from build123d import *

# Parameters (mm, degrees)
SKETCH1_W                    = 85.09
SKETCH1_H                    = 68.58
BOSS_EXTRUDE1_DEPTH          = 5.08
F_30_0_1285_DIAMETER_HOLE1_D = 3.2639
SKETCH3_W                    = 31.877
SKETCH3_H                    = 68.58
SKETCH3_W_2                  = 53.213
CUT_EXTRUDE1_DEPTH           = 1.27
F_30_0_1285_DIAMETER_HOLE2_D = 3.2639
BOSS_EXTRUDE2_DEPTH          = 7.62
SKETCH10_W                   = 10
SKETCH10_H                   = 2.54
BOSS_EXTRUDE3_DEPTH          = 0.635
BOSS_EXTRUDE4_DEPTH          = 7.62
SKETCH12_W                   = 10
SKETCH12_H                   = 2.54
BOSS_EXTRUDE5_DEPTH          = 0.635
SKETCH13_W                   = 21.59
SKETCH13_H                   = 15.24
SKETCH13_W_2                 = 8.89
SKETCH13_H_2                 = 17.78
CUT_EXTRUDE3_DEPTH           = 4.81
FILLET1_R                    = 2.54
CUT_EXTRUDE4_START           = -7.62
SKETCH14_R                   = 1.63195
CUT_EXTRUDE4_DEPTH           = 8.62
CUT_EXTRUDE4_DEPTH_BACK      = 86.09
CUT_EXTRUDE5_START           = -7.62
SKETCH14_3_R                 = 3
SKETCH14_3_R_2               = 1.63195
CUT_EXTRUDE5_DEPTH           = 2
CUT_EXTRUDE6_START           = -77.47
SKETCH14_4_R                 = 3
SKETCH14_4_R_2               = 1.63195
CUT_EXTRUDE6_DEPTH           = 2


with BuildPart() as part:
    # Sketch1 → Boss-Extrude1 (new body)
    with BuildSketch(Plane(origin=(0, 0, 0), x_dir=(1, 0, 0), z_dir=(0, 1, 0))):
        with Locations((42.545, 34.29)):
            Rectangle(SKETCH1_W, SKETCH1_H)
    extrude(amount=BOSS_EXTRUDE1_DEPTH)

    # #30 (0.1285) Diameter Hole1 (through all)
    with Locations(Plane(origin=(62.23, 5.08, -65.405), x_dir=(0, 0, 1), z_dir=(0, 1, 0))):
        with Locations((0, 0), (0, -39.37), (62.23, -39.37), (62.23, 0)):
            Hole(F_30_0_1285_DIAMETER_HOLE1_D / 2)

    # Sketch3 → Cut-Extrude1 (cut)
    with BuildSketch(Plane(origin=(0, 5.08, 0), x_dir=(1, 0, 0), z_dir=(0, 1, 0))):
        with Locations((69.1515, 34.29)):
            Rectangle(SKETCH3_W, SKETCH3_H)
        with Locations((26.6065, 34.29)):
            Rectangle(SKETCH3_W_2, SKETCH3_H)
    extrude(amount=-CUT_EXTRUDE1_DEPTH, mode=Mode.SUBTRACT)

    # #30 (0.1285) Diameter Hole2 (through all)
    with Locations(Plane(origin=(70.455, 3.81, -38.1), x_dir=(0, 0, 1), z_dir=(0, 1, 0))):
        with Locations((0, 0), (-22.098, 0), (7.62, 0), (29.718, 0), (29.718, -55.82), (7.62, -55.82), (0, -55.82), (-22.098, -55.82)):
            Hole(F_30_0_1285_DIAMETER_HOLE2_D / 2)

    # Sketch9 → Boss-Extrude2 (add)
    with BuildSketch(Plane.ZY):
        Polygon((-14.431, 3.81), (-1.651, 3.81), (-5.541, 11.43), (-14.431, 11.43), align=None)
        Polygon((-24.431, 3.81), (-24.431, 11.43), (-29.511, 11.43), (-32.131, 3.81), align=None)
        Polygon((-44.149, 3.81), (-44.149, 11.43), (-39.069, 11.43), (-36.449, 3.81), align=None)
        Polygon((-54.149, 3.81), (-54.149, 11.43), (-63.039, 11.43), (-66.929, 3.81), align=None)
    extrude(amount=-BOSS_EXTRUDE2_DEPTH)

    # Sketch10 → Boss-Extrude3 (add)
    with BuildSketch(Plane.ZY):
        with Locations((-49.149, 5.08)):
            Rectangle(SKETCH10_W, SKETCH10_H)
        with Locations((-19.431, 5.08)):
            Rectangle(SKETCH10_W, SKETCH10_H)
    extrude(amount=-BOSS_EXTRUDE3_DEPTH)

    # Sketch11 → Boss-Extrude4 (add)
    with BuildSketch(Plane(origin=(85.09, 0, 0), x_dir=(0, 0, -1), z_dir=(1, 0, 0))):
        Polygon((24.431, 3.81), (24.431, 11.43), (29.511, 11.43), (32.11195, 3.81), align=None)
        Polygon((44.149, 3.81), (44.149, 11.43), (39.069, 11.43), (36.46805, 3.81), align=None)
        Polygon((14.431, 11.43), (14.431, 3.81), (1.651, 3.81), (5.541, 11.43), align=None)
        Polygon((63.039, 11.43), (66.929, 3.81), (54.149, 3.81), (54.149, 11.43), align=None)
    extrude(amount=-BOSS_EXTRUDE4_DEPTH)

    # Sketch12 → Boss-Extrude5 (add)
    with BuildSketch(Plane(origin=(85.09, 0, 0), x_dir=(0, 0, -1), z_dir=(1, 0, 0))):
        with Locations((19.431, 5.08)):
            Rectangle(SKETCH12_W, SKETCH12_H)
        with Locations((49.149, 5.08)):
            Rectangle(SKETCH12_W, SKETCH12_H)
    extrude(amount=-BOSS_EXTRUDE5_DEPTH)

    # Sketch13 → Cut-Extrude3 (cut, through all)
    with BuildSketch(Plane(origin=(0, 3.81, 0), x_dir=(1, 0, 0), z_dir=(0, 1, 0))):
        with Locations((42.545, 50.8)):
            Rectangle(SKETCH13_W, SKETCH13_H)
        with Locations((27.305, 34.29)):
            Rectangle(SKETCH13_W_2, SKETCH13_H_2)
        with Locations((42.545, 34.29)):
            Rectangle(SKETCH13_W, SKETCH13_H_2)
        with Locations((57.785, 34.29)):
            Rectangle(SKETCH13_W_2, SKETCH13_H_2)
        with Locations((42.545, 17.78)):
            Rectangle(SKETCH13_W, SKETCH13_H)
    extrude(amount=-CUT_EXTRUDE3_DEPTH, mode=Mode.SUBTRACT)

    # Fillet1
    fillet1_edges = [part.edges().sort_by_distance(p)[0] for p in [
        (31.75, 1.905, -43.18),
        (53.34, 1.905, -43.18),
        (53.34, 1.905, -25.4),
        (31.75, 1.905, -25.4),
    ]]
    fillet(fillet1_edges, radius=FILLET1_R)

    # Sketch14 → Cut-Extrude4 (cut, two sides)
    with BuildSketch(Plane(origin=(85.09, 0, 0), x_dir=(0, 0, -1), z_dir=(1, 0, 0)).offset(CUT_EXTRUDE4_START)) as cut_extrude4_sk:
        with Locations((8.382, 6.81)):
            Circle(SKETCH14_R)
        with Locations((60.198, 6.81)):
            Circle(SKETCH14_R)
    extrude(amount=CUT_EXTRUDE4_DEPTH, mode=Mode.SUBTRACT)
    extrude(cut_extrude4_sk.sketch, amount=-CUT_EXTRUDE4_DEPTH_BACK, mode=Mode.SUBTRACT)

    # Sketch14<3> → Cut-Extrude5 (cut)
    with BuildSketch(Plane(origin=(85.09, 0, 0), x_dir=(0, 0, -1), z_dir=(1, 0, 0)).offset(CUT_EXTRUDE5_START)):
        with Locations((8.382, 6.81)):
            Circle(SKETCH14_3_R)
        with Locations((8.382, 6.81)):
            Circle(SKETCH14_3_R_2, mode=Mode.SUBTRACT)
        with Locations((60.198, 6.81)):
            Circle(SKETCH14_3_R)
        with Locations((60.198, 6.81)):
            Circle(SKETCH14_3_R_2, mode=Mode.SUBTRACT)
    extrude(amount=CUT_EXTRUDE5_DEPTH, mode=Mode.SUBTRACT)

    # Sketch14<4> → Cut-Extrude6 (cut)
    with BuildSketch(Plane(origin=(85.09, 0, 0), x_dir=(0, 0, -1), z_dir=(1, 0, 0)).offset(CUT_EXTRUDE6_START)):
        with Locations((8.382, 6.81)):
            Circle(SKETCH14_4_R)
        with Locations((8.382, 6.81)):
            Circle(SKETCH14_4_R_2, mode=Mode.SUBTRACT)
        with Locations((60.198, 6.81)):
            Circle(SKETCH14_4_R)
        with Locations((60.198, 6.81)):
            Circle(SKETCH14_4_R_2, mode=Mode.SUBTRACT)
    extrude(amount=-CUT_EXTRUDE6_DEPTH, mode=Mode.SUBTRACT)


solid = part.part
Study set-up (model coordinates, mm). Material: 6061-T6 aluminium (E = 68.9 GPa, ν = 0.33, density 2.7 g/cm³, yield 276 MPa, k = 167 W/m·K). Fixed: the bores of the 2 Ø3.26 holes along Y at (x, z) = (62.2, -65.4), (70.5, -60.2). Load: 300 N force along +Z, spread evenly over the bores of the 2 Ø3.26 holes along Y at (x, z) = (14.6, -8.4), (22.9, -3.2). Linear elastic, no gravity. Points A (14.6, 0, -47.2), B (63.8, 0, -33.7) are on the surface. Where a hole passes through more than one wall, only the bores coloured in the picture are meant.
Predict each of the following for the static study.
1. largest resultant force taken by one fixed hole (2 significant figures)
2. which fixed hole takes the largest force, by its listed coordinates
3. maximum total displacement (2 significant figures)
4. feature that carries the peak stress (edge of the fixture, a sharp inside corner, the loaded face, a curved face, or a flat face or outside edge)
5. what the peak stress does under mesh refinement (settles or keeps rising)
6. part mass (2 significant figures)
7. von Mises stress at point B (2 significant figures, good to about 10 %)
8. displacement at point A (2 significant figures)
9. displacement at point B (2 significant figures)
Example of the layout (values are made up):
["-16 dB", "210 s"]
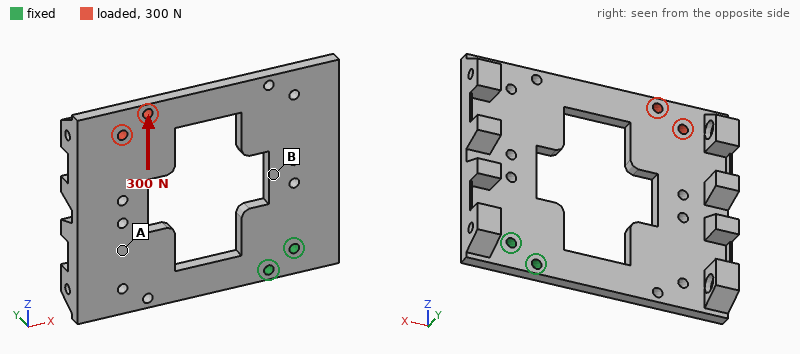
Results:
["1.2 kN", "(62.2, -65.4)", "0.13 mm", "edge of the fixture", "keeps rising", "55 g", "16 MPa", "0.088 mm", "0.026 mm"]
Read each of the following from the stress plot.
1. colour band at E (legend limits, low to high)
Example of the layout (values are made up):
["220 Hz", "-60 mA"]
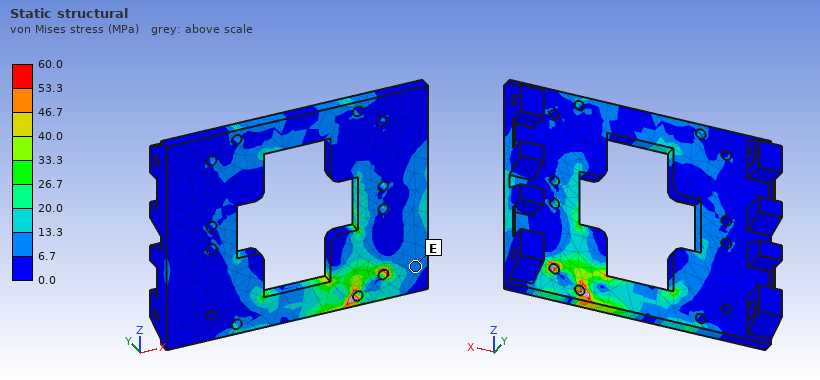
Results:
["6.7 to 13.3 MPa"]
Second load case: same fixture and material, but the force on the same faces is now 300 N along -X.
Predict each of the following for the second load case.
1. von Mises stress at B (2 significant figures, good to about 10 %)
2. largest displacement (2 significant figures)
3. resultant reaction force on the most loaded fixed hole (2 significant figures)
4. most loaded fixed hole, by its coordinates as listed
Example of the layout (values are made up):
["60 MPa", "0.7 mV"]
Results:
["13 MPa", "0.13 mm", "1.4 kN", "(70.5, -60.2)"]
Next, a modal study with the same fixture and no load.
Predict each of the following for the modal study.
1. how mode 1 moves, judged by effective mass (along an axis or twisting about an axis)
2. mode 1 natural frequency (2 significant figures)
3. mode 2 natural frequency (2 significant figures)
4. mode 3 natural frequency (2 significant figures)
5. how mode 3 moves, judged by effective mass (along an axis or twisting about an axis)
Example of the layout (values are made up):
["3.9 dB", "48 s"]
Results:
["along Y", "300 Hz", "670 Hz", "1300 Hz", "along Y"]
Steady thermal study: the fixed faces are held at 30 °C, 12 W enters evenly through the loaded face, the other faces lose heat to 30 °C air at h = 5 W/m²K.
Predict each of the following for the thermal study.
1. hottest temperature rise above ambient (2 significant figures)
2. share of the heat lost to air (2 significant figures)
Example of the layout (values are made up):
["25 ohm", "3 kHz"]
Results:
["53 K", "14 %"]
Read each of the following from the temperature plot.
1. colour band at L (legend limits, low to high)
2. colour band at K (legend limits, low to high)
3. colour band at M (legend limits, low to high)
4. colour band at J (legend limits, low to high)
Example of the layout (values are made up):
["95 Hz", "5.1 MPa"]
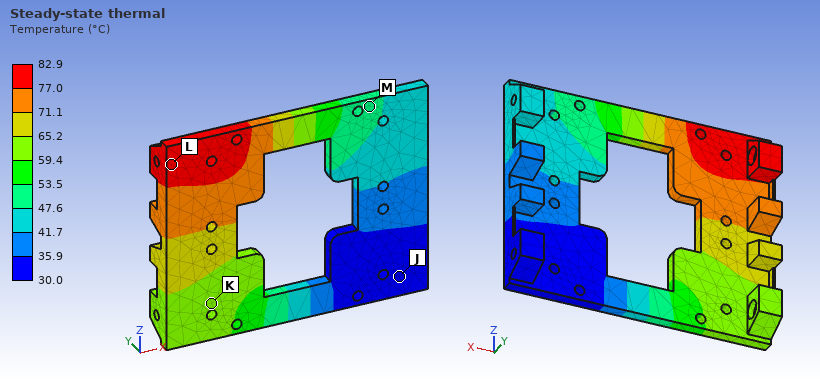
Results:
["77.0 to 82.9 °C", "59.4 to 65.2 °C", "47.6 to 53.5 °C", "30.0 to 35.9 °C"]
